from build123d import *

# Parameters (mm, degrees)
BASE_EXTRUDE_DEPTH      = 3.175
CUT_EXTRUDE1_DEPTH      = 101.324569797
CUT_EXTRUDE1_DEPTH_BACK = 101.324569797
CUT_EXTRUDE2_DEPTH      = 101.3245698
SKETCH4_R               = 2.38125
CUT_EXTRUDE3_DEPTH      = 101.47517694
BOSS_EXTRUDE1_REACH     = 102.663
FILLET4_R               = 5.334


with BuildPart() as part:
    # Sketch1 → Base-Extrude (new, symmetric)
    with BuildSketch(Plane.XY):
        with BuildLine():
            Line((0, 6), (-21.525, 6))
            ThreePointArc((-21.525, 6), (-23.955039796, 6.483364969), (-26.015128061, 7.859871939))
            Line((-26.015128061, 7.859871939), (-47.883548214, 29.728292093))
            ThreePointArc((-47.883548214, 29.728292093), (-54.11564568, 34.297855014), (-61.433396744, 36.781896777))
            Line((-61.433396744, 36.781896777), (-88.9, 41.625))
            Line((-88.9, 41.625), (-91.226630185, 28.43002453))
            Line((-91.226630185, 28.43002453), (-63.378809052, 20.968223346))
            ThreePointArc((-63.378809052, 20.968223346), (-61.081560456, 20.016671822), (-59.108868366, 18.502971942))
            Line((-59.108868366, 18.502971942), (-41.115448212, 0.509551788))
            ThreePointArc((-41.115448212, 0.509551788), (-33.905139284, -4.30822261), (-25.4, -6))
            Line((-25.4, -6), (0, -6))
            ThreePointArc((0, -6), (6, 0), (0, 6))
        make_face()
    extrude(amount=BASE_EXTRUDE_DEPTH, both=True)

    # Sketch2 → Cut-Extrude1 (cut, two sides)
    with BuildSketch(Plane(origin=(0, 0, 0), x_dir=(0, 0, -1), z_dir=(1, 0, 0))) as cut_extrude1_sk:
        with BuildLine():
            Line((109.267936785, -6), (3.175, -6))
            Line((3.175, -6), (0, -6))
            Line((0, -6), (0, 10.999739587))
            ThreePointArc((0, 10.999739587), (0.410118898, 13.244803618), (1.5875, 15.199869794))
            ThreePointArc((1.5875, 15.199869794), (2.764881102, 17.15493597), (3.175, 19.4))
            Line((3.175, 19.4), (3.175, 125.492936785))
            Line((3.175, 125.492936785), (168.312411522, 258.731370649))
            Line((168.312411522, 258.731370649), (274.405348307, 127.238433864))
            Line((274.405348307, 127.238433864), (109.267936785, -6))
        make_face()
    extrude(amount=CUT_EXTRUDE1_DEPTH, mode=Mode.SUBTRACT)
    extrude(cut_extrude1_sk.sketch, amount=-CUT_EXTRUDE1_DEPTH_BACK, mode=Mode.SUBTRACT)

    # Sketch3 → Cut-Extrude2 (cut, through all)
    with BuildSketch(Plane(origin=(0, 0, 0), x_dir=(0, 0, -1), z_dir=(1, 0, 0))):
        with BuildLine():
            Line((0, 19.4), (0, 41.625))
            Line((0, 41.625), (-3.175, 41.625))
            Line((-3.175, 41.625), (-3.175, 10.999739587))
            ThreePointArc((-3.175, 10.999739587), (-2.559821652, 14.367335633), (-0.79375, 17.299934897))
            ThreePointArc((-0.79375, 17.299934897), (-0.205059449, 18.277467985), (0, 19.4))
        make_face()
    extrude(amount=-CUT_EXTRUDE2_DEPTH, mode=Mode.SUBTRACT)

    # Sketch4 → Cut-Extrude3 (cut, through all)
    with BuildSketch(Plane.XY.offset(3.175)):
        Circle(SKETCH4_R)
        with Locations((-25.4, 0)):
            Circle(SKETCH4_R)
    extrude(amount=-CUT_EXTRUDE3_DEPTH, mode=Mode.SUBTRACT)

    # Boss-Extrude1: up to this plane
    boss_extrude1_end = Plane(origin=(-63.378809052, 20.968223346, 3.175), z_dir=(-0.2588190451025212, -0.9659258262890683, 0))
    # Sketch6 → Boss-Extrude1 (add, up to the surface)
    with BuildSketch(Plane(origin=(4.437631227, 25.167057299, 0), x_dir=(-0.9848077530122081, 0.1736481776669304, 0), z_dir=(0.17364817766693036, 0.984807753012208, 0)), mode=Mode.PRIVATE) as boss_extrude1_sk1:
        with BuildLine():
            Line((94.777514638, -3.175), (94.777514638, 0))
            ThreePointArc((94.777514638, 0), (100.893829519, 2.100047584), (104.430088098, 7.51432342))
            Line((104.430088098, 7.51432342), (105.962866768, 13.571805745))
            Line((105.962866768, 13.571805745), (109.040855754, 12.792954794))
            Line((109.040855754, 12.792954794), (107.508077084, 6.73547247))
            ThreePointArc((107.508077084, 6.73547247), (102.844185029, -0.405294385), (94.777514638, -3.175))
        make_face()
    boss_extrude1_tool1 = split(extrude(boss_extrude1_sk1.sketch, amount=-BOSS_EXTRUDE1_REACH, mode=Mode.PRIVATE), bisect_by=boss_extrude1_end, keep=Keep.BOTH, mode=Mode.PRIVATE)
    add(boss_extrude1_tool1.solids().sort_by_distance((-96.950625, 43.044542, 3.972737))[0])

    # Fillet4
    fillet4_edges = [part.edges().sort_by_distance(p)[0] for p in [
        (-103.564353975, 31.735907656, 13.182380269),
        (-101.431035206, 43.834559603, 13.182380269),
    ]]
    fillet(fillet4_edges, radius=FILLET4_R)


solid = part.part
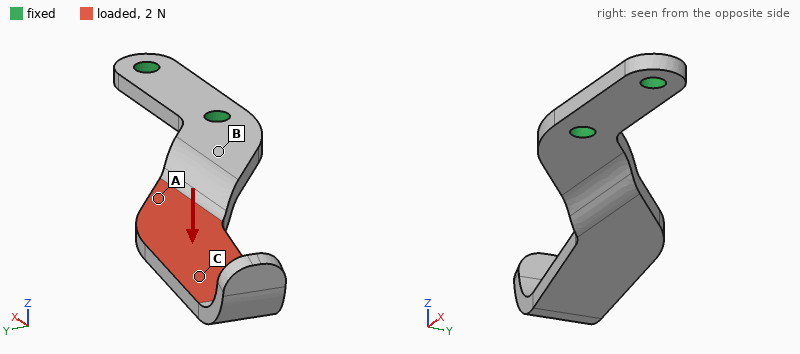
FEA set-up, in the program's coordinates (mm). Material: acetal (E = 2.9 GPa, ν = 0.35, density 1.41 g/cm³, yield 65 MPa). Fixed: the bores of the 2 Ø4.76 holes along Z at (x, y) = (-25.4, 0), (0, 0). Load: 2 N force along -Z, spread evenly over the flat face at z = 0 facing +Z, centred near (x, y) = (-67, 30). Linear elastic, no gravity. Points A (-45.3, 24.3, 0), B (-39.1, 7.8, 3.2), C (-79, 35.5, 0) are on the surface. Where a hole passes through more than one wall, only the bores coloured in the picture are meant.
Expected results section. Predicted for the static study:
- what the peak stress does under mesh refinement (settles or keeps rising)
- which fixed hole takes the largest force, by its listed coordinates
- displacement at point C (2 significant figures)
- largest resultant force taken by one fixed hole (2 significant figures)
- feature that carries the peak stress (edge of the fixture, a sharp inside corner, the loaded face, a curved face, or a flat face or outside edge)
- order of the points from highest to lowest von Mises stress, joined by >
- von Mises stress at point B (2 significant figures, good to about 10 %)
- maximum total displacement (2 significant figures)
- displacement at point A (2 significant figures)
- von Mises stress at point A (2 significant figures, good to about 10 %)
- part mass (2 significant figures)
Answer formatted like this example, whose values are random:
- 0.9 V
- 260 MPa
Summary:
- keeps rising
- (-25.4, 0)
- 0.95 mm
- 2.2 N
- edge of the fixture
- B > A > C
- 2.5 MPa
- 1.5 mm
- 0.29 mm
- 1.4 MPa
- 7.9 g
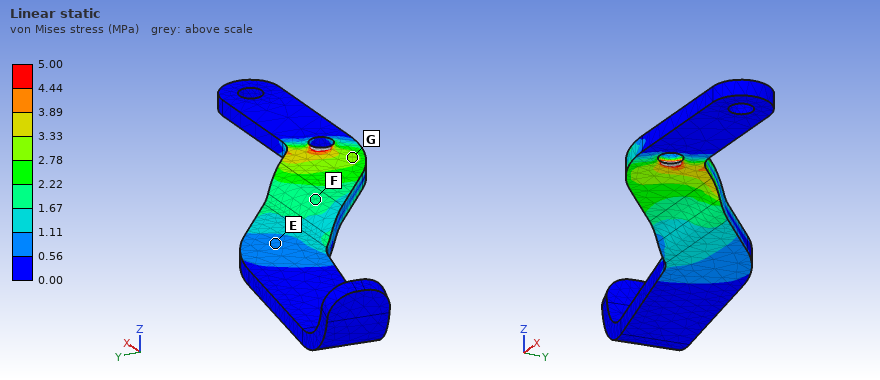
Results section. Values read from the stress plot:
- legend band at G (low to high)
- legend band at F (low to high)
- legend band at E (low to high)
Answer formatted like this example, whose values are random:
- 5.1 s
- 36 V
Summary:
- 2.78 to 3.33 MPa
- 1.67 to 2.22 MPa
- 0.56 to 1.11 MPa
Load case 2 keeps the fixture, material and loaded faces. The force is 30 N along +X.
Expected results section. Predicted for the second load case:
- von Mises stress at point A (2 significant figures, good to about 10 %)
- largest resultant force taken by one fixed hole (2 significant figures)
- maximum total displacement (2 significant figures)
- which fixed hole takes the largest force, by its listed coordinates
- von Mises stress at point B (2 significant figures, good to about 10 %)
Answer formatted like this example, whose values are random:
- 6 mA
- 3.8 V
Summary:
- 4.5 MPa
- 26 N
- 1.1 mm
- (-25.4, 0)
- 1.2 MPa
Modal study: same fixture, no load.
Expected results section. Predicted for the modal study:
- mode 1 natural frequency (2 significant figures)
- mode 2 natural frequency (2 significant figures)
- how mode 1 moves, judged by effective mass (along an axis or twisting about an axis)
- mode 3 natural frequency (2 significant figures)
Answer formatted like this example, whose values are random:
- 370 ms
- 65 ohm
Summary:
- 95 Hz
- 340 Hz
- along Z
- 480 Hz
